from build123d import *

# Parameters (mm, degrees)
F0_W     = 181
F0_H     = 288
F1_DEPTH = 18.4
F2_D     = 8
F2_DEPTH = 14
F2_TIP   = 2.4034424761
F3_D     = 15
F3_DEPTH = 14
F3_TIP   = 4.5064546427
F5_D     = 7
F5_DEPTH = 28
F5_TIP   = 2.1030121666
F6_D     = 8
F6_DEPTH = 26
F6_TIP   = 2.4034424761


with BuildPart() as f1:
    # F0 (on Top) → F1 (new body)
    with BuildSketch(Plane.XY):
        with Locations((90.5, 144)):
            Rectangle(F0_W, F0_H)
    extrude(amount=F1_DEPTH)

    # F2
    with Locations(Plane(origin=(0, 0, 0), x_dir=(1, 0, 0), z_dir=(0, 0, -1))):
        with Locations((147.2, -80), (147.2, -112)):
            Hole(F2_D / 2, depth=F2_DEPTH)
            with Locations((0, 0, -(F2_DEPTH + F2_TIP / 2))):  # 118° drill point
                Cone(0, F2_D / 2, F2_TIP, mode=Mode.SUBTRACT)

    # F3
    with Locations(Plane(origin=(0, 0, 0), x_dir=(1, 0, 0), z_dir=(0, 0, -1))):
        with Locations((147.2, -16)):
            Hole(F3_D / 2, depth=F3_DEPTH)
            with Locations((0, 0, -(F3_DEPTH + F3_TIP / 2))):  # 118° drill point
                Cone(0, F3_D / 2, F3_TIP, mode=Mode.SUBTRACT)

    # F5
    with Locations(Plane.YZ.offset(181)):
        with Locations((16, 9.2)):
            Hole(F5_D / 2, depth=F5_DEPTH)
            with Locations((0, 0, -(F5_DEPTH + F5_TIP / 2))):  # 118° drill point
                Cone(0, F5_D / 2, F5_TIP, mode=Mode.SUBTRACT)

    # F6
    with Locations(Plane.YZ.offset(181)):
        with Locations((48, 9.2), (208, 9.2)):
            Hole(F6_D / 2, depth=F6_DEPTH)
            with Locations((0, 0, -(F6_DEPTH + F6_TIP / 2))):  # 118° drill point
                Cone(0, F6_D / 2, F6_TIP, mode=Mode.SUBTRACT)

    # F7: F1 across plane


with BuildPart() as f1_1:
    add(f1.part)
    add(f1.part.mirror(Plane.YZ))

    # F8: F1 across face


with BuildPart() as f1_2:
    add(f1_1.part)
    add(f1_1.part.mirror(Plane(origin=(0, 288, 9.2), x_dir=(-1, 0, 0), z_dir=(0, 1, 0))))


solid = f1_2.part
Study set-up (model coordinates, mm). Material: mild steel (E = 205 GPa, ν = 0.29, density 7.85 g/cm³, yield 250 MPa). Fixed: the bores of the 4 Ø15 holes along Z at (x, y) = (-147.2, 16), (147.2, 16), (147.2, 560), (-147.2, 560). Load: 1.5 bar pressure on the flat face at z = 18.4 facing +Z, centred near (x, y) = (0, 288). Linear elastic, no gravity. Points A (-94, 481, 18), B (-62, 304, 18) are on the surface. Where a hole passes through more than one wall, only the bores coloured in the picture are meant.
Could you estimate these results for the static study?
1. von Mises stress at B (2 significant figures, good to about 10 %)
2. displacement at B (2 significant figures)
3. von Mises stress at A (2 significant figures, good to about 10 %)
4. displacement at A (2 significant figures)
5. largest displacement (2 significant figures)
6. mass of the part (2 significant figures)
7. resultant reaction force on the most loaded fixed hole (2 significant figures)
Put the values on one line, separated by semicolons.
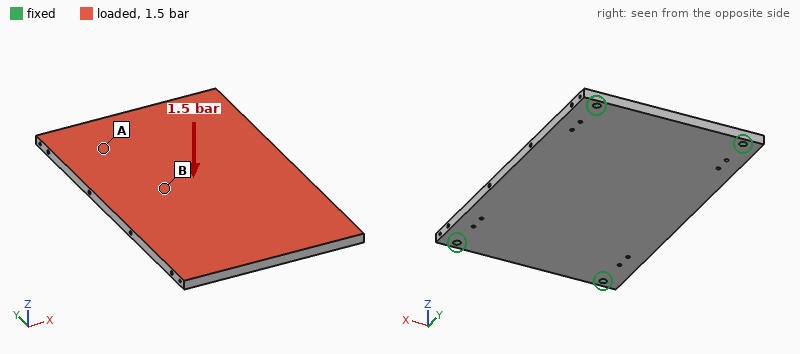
38 MPa; 0.52 mm; 12 MPa; 0.20 mm; 0.53 mm; 30 kg; 8.0 kN
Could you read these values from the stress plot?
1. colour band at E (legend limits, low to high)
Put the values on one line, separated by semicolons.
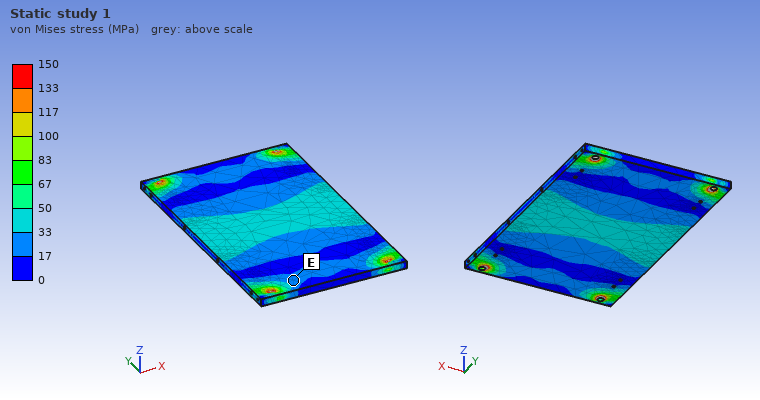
17 to 33 MPa
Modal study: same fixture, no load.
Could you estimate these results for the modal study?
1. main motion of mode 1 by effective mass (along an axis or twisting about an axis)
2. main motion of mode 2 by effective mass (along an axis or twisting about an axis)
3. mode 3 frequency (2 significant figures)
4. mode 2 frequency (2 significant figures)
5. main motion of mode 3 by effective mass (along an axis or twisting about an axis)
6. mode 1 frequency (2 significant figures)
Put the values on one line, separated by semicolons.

along Z; twisting about Y; 690 Hz; 440 Hz; twisting about X; 250 Hz
